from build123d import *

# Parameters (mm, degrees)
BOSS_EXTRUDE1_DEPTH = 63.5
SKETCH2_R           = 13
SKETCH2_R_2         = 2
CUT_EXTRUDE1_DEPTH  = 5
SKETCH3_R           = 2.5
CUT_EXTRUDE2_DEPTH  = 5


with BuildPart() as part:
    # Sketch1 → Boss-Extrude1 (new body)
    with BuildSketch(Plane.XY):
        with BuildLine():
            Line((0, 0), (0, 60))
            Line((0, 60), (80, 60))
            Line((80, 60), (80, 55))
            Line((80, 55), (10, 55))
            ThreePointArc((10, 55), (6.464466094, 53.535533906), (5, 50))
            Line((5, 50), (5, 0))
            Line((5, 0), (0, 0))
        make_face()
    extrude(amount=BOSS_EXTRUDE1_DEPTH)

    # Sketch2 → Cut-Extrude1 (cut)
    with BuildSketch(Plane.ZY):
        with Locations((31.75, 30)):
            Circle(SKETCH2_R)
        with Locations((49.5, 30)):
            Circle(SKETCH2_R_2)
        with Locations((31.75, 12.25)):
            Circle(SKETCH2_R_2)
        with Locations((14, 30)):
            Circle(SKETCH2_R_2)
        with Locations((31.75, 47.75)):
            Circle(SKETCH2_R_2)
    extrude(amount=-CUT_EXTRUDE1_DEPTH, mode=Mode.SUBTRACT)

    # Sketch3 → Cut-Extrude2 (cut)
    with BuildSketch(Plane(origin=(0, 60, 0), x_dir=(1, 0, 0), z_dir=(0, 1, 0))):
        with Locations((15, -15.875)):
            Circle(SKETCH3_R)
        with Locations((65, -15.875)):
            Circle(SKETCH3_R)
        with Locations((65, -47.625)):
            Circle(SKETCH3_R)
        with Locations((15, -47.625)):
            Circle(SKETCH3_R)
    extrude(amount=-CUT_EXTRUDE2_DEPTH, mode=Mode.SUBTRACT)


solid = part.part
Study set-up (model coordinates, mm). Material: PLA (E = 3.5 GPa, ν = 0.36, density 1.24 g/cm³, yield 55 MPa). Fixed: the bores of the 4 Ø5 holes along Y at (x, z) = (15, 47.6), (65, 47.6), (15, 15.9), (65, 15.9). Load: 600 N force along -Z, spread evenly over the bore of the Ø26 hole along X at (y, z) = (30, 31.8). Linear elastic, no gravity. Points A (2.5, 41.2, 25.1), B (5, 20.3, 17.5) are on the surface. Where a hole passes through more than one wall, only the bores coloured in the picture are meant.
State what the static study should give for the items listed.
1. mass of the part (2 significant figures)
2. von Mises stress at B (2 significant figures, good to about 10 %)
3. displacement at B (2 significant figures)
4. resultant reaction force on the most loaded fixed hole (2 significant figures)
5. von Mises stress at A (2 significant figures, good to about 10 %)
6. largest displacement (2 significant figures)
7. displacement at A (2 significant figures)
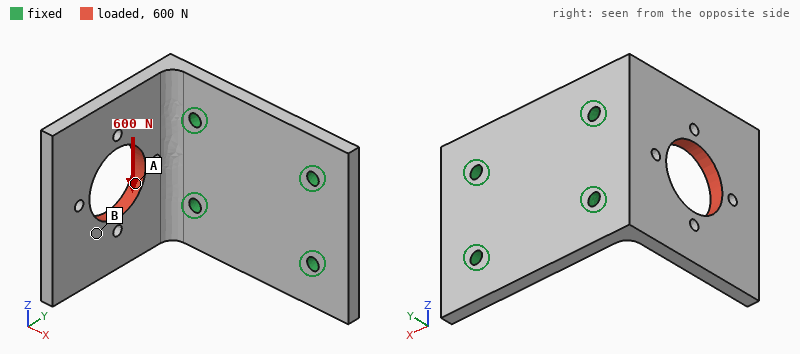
49 g
5.2 MPa
0.62 mm
570 N
12 MPa
1.0 mm
0.23 mm
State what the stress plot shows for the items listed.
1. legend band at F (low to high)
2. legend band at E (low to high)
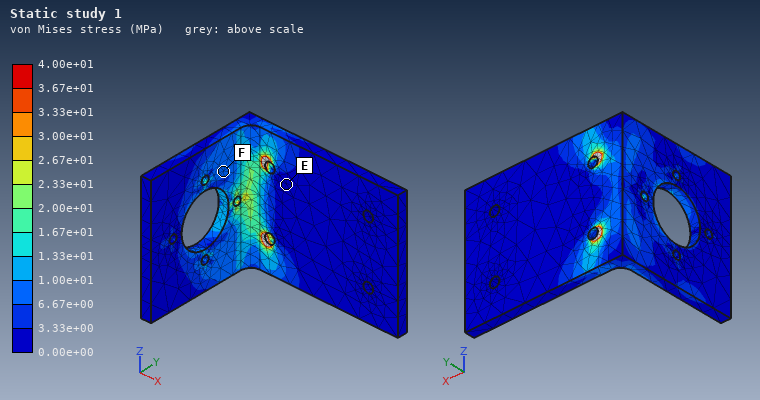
6.67e+00 to 1.00e+01 MPa
0.00e+00 to 3.33e+00 MPa
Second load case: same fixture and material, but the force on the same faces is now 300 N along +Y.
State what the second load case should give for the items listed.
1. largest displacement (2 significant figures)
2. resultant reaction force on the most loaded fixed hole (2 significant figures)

0.61 mm
160 N
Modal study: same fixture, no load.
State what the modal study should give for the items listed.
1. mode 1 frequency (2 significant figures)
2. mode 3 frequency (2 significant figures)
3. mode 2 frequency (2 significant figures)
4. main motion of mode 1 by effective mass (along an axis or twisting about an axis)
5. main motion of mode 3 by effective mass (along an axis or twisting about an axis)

330 Hz
1100 Hz
730 Hz
along X
along Z
